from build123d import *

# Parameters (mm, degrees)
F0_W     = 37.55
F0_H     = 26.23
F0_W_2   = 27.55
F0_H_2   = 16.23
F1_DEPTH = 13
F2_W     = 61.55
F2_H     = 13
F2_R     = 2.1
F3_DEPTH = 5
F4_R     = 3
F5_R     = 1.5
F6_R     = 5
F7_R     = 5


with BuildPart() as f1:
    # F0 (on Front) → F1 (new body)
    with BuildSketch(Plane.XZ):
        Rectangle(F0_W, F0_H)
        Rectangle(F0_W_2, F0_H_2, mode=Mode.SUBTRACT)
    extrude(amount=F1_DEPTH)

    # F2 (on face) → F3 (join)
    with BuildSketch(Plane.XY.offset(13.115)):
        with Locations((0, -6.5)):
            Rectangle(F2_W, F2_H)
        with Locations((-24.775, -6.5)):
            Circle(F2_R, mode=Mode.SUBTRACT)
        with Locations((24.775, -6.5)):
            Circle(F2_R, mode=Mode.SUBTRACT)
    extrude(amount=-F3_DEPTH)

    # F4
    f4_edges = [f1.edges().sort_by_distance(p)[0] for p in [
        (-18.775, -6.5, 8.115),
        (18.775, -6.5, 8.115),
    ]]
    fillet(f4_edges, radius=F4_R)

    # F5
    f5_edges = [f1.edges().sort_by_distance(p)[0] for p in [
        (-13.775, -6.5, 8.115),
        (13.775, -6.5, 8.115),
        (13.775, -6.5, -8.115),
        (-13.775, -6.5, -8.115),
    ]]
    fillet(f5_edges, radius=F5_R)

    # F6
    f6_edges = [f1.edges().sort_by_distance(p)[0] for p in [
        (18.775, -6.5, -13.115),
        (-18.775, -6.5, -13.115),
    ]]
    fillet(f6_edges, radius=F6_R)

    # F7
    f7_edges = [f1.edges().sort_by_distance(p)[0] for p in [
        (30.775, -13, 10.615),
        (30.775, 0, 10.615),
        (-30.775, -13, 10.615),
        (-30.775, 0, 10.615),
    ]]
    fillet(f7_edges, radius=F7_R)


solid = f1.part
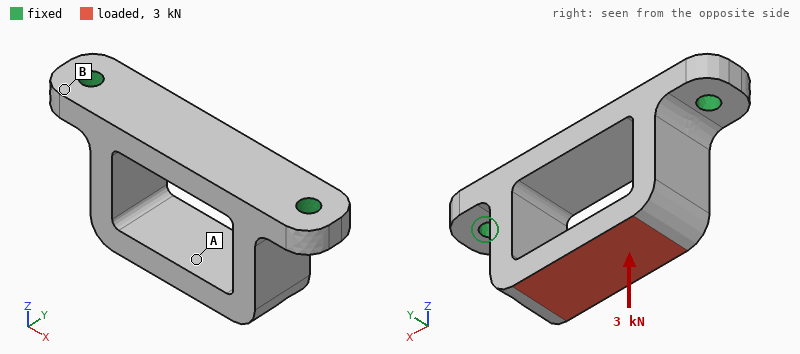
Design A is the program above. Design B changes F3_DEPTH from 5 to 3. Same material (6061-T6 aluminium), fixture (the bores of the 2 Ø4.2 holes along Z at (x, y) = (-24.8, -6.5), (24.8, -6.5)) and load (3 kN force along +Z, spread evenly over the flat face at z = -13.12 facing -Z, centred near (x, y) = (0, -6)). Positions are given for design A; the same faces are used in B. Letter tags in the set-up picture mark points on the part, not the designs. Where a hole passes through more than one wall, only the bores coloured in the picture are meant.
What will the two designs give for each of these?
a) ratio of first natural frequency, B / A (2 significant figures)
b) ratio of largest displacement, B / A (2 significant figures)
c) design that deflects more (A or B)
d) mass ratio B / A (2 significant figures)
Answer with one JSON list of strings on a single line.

["0.62", "1.2", "B", "0.94"]
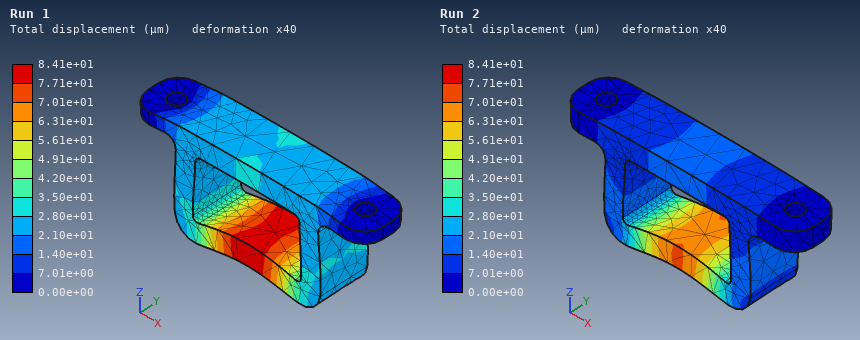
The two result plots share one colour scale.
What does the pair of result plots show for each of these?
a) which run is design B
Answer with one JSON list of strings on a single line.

["Run 1"]
